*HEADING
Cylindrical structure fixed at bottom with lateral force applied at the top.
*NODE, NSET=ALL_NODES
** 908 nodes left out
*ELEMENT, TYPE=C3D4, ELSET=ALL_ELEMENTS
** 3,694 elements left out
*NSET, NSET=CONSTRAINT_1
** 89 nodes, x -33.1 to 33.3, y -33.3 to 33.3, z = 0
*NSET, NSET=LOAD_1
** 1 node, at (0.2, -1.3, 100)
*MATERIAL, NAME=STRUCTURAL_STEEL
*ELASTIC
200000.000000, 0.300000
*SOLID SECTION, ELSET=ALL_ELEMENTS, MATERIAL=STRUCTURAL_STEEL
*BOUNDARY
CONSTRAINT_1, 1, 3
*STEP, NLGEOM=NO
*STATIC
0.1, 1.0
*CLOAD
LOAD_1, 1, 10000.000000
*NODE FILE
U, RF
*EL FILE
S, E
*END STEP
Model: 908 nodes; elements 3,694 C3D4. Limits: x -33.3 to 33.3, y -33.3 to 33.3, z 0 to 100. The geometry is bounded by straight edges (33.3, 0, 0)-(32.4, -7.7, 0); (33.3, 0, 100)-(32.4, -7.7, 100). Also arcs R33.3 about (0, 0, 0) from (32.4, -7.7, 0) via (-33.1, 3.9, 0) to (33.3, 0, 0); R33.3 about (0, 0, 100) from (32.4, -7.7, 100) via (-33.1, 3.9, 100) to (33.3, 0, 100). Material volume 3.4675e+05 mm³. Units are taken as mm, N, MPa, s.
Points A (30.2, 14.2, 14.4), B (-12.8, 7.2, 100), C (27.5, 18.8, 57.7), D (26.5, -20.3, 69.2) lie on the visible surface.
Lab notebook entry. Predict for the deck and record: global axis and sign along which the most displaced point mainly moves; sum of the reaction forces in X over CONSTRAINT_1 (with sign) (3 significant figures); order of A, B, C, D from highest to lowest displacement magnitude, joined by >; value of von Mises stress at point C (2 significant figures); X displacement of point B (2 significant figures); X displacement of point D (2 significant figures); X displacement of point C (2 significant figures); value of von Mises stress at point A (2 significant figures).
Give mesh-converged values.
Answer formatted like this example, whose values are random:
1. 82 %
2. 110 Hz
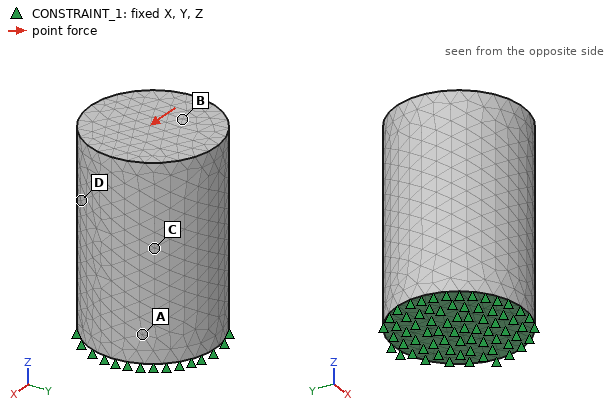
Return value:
1. +X
2. -10000 N
3. B > D > C > A
4. 12 MPa
5. 0.021 mm
6. 0.012 mm
7. 0.0092 mm
8. 25 MPa
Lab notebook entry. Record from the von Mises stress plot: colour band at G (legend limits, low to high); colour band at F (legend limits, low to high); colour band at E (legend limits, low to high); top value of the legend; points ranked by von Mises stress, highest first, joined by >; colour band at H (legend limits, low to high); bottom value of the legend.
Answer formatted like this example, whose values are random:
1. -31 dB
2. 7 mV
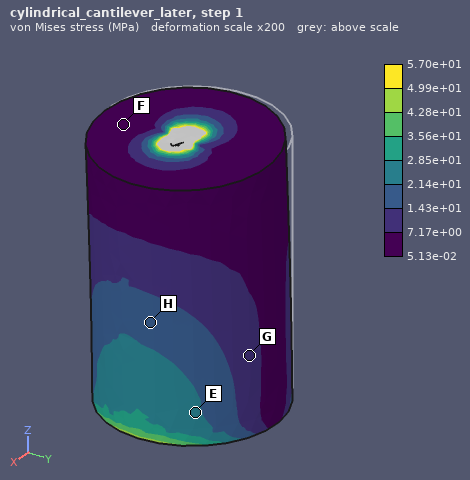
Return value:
1. 7.17e+00 to 1.43e+01 MPa
2. 5.13e-02 to 7.17e+00 MPa
3. 2.14e+01 to 2.85e+01 MPa
4. 5.70e+01 MPa
5. E > H > G > F
6. 1.43e+01 to 2.14e+01 MPa
7. 5.13e-02 MPa
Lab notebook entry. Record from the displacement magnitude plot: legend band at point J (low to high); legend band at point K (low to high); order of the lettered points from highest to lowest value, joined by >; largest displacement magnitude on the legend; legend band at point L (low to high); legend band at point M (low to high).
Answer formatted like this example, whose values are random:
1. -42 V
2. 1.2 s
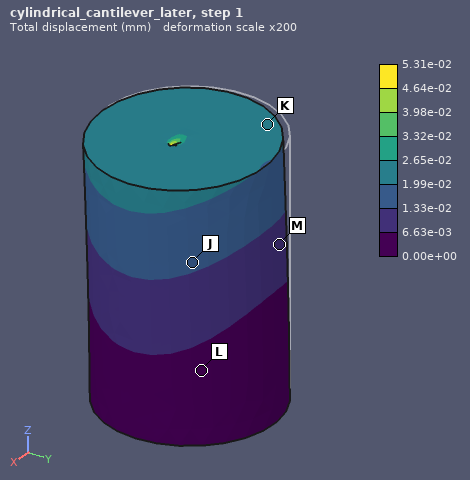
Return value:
1. 1.33e-02 to 1.99e-02 mm
2. 1.99e-02 to 2.65e-02 mm
3. K > J > M > L
4. 5.31e-02 mm
5. 0.00e+00 to 6.63e-03 mm
6. 6.63e-03 to 1.33e-02 mm
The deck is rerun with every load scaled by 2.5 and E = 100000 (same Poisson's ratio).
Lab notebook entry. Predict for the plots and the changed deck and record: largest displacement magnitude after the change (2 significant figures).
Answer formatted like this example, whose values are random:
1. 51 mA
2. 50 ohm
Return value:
1. 0.27 mm
